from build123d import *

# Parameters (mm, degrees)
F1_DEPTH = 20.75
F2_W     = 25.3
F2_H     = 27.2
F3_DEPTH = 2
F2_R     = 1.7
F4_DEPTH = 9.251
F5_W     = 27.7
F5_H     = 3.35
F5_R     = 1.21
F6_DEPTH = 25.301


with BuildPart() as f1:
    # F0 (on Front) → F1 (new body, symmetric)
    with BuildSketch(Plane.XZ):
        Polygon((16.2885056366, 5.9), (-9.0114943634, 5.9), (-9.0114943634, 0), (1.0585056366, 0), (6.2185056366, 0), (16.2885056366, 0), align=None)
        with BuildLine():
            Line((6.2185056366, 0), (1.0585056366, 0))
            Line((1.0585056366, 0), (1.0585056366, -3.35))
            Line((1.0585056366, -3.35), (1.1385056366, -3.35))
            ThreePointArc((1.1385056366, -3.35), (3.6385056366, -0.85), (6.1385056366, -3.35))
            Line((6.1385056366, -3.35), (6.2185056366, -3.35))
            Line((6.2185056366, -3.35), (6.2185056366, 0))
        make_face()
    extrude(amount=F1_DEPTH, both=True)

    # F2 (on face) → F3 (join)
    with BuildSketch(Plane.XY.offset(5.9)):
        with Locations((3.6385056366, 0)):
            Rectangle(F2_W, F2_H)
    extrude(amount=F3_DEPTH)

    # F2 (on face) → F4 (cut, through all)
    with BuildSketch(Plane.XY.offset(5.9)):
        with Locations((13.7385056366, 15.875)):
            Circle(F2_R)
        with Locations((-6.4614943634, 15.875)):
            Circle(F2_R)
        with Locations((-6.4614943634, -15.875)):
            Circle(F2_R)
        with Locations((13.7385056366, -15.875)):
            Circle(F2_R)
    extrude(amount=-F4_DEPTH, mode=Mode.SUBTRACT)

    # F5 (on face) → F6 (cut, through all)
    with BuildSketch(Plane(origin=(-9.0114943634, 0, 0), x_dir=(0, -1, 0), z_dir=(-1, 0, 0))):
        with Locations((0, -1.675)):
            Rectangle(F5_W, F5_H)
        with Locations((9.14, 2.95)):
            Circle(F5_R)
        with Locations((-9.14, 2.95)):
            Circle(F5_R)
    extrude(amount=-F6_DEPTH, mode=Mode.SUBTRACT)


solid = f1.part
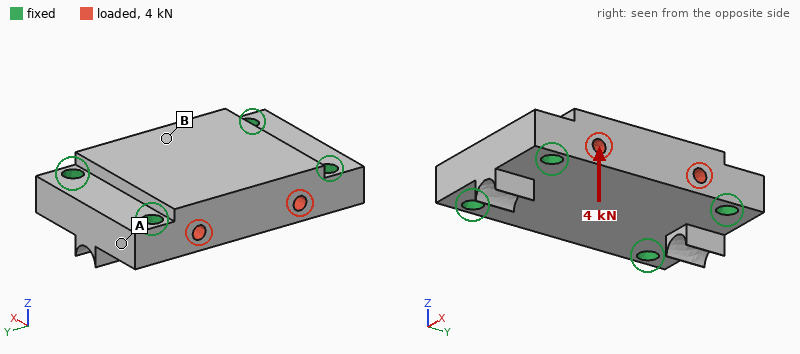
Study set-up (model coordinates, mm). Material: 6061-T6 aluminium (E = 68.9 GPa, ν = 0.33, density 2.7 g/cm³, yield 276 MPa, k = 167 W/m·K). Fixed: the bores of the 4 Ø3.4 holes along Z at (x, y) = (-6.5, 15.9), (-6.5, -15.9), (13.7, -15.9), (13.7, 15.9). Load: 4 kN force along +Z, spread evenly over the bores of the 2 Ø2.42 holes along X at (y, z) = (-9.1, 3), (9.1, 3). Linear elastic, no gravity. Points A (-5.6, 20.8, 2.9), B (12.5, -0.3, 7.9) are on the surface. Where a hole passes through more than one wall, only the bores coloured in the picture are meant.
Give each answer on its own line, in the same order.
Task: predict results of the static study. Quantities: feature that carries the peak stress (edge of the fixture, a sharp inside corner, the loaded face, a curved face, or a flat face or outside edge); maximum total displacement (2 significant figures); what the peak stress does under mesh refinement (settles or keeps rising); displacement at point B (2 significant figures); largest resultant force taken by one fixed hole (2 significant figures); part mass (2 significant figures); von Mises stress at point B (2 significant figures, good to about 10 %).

edge of the fixture
12 µm
keeps rising
11 µm
1.0 kN
20 g
23 MPa
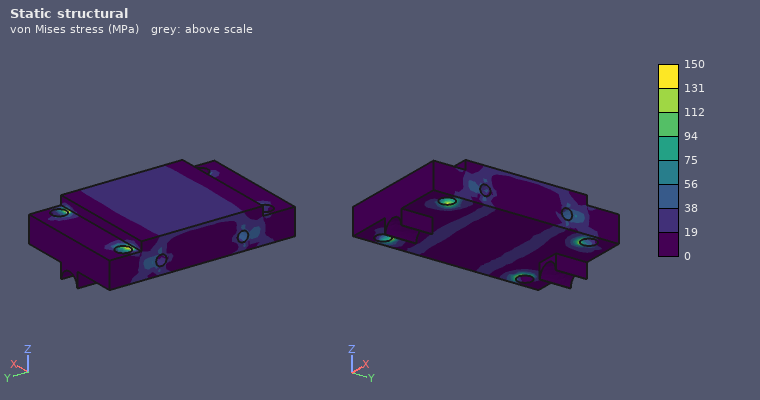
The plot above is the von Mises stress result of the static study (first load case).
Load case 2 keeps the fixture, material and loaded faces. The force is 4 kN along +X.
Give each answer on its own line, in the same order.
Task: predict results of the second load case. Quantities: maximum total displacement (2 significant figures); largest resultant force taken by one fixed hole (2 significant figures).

4.7 µm
1.1 kN
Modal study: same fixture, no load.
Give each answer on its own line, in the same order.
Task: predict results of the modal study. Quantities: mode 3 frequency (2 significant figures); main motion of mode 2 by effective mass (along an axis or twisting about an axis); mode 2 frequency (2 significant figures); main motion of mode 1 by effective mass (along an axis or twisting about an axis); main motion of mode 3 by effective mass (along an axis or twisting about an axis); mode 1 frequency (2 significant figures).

39 kHz
twisting about Y
33 kHz
along Z
along X
24 kHz
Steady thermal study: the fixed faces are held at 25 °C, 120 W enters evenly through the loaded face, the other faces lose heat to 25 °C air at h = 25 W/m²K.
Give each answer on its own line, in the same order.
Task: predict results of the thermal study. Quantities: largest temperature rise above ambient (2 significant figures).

20 K
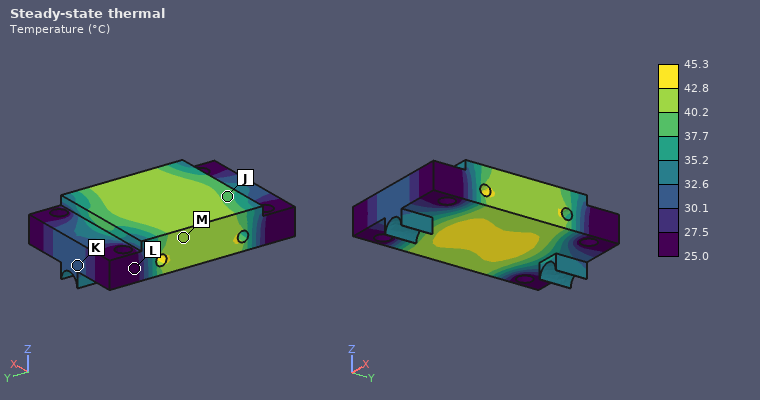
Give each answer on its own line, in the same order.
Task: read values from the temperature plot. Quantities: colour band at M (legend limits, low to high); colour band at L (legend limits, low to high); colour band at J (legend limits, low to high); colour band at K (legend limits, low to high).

40.2 to 42.8 °C
25.0 to 27.5 °C
37.7 to 40.2 °C
30.1 to 32.6 °C
